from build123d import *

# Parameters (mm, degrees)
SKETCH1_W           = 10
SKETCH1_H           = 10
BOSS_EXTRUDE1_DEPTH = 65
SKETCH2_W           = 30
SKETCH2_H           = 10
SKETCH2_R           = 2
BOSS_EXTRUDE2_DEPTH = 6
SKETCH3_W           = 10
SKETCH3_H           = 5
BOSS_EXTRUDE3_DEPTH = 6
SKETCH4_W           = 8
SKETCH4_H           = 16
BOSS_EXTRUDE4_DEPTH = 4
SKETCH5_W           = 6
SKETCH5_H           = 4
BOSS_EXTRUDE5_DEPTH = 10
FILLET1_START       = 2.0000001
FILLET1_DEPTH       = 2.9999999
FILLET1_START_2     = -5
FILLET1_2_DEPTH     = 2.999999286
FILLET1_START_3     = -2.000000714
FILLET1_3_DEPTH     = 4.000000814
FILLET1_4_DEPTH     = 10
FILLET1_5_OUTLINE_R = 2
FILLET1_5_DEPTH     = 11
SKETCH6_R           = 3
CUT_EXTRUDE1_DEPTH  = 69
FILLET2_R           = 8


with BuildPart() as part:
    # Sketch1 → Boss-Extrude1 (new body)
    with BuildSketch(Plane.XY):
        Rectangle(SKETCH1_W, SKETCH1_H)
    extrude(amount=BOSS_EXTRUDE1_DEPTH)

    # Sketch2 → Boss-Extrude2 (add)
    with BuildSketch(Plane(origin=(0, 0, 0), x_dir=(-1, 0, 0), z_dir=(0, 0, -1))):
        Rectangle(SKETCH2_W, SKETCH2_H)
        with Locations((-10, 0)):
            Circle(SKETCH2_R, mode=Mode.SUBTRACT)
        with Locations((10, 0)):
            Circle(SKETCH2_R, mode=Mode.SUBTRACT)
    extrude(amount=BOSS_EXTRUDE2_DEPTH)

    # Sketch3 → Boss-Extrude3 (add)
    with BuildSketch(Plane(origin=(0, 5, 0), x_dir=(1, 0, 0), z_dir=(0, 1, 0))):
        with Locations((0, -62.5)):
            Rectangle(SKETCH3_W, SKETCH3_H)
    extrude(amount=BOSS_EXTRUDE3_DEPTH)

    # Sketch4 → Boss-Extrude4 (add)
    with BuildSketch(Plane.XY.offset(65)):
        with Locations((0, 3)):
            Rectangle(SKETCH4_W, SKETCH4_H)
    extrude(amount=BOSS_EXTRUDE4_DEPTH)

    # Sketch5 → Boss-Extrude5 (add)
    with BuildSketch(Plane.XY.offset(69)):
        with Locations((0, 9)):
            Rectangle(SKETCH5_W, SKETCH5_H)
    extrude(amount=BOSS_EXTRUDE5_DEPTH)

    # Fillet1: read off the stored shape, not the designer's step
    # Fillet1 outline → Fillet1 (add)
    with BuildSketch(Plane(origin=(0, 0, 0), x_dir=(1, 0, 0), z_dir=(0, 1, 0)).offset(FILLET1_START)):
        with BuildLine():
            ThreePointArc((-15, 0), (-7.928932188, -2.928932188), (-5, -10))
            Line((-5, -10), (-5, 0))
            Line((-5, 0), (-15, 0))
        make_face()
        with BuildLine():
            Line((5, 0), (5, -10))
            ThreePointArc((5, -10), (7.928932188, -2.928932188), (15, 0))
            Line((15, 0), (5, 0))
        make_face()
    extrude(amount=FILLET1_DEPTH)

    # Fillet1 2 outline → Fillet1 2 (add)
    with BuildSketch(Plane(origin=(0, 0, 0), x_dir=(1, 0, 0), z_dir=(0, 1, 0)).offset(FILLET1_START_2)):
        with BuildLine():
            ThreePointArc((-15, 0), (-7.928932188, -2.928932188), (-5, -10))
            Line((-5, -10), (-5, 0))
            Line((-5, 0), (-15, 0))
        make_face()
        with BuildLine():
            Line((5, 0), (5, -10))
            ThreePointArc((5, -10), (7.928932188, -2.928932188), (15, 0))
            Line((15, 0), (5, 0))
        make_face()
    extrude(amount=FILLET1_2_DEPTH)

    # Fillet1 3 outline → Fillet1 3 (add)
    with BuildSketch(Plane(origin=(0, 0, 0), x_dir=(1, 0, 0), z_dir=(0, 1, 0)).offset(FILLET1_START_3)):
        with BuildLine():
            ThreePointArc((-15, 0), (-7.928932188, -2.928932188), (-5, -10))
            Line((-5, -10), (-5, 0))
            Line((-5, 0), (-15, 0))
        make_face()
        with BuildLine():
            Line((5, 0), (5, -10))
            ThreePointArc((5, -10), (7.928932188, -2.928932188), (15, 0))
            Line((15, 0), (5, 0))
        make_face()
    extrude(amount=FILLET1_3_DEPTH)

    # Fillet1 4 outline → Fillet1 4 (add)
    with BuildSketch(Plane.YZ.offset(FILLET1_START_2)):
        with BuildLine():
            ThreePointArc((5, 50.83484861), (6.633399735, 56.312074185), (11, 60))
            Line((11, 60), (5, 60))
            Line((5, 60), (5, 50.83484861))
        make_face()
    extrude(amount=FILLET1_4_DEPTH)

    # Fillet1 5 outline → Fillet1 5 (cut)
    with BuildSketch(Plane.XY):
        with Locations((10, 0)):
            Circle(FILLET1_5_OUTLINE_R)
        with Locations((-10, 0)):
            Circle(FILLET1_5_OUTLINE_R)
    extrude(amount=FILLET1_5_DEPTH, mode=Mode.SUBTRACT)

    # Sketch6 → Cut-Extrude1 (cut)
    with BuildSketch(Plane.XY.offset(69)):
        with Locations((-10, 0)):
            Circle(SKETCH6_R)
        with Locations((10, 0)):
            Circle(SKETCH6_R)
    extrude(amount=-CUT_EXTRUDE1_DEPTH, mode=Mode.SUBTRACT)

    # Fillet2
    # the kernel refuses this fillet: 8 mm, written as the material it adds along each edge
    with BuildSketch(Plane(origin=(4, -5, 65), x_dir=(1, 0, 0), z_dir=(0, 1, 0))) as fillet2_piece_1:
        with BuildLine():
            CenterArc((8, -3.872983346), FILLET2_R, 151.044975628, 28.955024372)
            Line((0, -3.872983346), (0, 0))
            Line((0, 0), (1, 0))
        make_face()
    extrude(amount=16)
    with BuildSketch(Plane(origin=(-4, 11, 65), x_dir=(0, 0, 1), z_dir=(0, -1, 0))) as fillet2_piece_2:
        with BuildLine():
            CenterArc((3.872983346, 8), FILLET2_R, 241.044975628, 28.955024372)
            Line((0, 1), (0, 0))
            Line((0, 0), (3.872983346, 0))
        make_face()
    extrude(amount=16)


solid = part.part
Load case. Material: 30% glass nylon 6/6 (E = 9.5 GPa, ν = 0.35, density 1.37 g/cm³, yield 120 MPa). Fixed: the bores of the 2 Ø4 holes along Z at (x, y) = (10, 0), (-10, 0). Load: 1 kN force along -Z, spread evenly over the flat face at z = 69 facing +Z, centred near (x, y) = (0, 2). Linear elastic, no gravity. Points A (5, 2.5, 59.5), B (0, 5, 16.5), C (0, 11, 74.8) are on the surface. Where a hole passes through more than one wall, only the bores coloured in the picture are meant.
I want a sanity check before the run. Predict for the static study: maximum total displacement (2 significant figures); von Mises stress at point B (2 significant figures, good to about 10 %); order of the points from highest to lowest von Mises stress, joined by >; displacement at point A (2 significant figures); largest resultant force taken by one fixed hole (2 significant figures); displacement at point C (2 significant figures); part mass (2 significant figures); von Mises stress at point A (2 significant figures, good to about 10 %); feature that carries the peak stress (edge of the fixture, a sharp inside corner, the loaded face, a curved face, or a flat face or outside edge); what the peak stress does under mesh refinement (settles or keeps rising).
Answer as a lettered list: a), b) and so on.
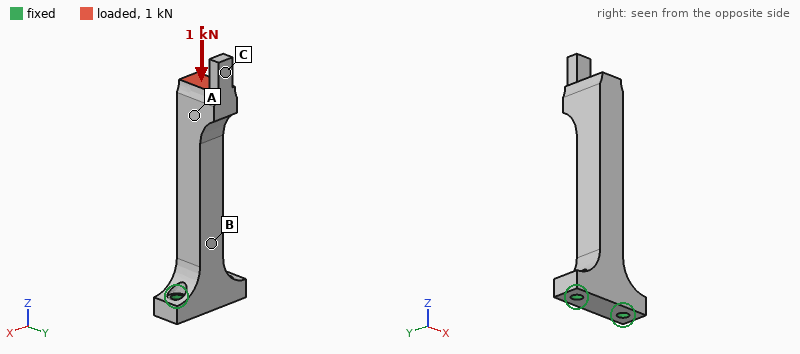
a) 0.70 mm
b) 20 MPa
c) B > A > C
d) 0.44 mm
e) 540 N
f) 0.65 mm
g) 13 g
h) 9.8 MPa
i) edge of the fixture
j) keeps rising
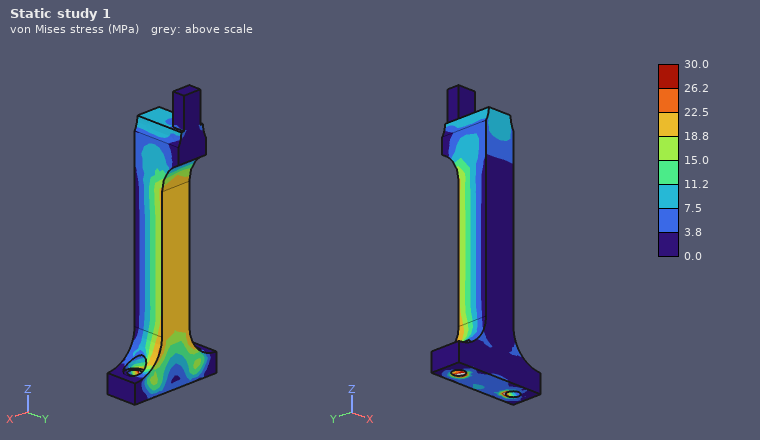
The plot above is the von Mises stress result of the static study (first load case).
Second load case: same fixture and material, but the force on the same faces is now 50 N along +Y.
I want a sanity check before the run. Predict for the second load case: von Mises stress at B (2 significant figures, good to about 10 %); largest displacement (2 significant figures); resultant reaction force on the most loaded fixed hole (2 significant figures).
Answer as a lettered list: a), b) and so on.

a) 16 MPa
b) 1.1 mm
c) 25 N
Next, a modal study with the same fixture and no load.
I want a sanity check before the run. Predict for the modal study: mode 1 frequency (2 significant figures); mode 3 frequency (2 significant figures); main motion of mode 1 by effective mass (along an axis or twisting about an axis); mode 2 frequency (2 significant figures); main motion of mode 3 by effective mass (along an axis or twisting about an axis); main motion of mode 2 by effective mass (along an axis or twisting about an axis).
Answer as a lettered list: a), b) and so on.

a) 640 Hz
b) 3800 Hz
c) along Y
d) 790 Hz
e) along Y
f) along X
